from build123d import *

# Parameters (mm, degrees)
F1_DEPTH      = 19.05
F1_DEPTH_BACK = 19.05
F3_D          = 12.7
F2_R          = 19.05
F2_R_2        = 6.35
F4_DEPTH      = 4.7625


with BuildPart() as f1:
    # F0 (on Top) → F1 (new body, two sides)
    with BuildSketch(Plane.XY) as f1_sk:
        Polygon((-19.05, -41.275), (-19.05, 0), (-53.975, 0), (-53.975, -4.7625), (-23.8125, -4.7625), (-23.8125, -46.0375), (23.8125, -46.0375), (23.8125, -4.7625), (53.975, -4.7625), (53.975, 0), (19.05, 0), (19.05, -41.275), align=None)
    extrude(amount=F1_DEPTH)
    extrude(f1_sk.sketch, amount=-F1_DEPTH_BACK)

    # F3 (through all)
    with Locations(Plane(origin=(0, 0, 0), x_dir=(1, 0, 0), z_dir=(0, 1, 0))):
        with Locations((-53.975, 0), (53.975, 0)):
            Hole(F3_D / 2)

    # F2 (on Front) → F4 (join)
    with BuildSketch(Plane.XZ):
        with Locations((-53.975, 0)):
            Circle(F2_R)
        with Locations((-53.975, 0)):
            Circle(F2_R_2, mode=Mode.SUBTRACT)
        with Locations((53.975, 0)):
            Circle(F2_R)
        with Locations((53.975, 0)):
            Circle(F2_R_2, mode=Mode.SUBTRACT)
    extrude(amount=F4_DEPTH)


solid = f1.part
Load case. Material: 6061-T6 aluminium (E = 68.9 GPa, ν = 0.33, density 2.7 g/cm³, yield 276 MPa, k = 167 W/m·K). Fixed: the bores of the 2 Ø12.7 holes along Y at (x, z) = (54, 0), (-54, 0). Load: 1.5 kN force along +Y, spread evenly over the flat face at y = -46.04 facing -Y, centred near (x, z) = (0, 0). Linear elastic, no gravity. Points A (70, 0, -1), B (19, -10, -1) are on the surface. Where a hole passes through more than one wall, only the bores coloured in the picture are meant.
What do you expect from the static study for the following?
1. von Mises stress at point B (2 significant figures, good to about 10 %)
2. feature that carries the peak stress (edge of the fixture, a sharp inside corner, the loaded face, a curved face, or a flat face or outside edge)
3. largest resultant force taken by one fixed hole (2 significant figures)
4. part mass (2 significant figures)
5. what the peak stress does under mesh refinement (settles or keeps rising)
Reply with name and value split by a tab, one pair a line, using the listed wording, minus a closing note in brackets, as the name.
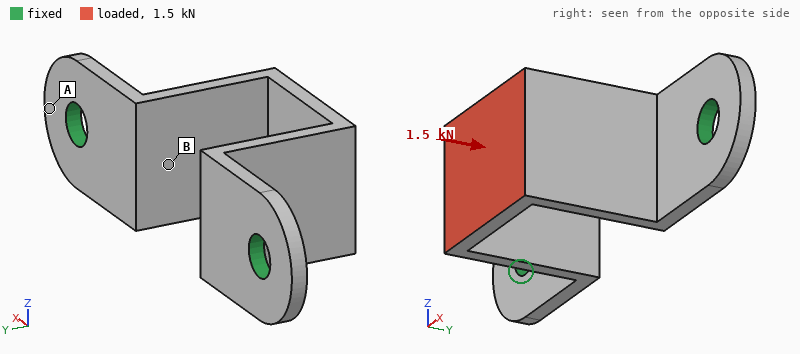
von Mises stress at point B	33 MPa
feature that carries the peak stress	edge of the fixture
largest resultant force taken by one fixed hole	820 N
part mass	100 g
what the peak stress does under mesh refinement	keeps rising
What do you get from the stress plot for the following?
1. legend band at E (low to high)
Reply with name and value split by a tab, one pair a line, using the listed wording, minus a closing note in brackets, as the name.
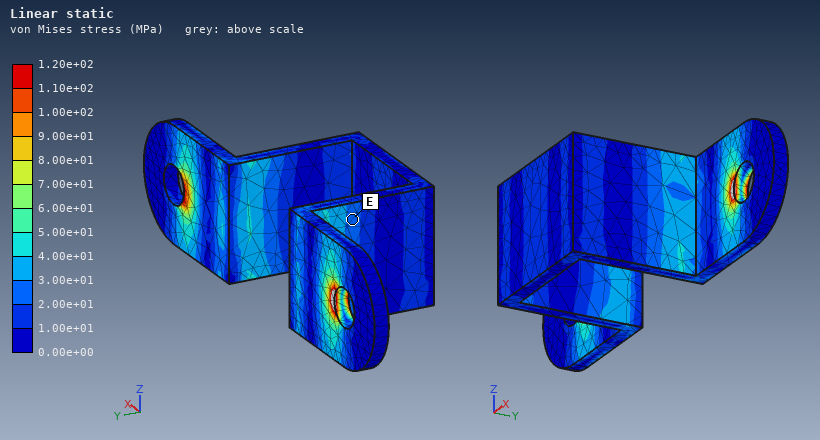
legend band at E	2.00e+01 to 3.00e+01 MPa
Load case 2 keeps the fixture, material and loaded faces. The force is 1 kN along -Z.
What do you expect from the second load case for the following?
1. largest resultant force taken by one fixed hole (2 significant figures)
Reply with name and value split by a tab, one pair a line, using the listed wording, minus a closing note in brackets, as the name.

largest resultant force taken by one fixed hole	500 N
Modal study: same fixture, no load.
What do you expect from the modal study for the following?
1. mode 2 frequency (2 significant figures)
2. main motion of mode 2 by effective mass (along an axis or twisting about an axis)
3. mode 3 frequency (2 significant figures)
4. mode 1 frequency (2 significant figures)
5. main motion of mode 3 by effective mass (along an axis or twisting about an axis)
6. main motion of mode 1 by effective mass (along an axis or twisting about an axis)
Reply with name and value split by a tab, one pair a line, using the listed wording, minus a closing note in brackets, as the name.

mode 2 frequency	1800 Hz
main motion of mode 2 by effective mass	along X
mode 3 frequency	2200 Hz
mode 1 frequency	1100 Hz
main motion of mode 3 by effective mass	along Y
main motion of mode 1 by effective mass	along Z
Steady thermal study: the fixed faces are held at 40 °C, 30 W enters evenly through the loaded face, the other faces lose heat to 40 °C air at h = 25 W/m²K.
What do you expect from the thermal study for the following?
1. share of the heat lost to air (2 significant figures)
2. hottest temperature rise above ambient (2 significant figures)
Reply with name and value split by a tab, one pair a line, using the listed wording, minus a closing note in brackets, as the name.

share of the heat lost to air	20 %
hottest temperature rise above ambient	33 K
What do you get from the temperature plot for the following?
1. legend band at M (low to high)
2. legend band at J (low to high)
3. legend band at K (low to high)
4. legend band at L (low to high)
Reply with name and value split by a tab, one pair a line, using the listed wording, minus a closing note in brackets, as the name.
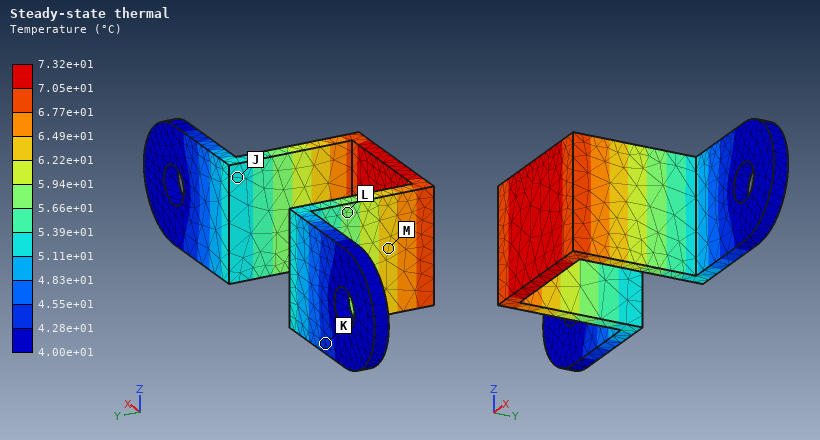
legend band at M	6.22e+01 to 6.49e+01 °C
legend band at J	5.11e+01 to 5.39e+01 °C
legend band at K	4.28e+01 to 4.55e+01 °C
legend band at L	5.66e+01 to 5.94e+01 °C
